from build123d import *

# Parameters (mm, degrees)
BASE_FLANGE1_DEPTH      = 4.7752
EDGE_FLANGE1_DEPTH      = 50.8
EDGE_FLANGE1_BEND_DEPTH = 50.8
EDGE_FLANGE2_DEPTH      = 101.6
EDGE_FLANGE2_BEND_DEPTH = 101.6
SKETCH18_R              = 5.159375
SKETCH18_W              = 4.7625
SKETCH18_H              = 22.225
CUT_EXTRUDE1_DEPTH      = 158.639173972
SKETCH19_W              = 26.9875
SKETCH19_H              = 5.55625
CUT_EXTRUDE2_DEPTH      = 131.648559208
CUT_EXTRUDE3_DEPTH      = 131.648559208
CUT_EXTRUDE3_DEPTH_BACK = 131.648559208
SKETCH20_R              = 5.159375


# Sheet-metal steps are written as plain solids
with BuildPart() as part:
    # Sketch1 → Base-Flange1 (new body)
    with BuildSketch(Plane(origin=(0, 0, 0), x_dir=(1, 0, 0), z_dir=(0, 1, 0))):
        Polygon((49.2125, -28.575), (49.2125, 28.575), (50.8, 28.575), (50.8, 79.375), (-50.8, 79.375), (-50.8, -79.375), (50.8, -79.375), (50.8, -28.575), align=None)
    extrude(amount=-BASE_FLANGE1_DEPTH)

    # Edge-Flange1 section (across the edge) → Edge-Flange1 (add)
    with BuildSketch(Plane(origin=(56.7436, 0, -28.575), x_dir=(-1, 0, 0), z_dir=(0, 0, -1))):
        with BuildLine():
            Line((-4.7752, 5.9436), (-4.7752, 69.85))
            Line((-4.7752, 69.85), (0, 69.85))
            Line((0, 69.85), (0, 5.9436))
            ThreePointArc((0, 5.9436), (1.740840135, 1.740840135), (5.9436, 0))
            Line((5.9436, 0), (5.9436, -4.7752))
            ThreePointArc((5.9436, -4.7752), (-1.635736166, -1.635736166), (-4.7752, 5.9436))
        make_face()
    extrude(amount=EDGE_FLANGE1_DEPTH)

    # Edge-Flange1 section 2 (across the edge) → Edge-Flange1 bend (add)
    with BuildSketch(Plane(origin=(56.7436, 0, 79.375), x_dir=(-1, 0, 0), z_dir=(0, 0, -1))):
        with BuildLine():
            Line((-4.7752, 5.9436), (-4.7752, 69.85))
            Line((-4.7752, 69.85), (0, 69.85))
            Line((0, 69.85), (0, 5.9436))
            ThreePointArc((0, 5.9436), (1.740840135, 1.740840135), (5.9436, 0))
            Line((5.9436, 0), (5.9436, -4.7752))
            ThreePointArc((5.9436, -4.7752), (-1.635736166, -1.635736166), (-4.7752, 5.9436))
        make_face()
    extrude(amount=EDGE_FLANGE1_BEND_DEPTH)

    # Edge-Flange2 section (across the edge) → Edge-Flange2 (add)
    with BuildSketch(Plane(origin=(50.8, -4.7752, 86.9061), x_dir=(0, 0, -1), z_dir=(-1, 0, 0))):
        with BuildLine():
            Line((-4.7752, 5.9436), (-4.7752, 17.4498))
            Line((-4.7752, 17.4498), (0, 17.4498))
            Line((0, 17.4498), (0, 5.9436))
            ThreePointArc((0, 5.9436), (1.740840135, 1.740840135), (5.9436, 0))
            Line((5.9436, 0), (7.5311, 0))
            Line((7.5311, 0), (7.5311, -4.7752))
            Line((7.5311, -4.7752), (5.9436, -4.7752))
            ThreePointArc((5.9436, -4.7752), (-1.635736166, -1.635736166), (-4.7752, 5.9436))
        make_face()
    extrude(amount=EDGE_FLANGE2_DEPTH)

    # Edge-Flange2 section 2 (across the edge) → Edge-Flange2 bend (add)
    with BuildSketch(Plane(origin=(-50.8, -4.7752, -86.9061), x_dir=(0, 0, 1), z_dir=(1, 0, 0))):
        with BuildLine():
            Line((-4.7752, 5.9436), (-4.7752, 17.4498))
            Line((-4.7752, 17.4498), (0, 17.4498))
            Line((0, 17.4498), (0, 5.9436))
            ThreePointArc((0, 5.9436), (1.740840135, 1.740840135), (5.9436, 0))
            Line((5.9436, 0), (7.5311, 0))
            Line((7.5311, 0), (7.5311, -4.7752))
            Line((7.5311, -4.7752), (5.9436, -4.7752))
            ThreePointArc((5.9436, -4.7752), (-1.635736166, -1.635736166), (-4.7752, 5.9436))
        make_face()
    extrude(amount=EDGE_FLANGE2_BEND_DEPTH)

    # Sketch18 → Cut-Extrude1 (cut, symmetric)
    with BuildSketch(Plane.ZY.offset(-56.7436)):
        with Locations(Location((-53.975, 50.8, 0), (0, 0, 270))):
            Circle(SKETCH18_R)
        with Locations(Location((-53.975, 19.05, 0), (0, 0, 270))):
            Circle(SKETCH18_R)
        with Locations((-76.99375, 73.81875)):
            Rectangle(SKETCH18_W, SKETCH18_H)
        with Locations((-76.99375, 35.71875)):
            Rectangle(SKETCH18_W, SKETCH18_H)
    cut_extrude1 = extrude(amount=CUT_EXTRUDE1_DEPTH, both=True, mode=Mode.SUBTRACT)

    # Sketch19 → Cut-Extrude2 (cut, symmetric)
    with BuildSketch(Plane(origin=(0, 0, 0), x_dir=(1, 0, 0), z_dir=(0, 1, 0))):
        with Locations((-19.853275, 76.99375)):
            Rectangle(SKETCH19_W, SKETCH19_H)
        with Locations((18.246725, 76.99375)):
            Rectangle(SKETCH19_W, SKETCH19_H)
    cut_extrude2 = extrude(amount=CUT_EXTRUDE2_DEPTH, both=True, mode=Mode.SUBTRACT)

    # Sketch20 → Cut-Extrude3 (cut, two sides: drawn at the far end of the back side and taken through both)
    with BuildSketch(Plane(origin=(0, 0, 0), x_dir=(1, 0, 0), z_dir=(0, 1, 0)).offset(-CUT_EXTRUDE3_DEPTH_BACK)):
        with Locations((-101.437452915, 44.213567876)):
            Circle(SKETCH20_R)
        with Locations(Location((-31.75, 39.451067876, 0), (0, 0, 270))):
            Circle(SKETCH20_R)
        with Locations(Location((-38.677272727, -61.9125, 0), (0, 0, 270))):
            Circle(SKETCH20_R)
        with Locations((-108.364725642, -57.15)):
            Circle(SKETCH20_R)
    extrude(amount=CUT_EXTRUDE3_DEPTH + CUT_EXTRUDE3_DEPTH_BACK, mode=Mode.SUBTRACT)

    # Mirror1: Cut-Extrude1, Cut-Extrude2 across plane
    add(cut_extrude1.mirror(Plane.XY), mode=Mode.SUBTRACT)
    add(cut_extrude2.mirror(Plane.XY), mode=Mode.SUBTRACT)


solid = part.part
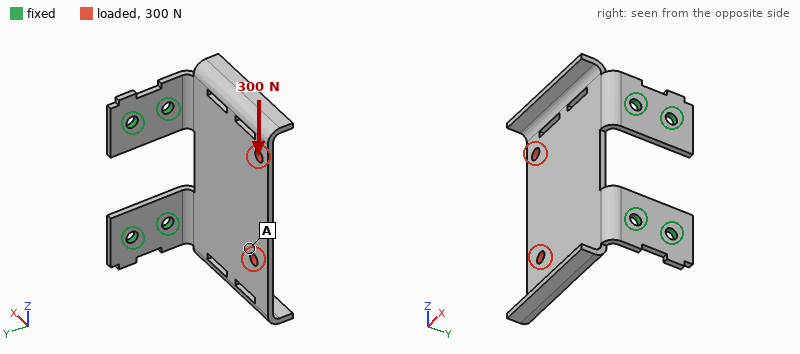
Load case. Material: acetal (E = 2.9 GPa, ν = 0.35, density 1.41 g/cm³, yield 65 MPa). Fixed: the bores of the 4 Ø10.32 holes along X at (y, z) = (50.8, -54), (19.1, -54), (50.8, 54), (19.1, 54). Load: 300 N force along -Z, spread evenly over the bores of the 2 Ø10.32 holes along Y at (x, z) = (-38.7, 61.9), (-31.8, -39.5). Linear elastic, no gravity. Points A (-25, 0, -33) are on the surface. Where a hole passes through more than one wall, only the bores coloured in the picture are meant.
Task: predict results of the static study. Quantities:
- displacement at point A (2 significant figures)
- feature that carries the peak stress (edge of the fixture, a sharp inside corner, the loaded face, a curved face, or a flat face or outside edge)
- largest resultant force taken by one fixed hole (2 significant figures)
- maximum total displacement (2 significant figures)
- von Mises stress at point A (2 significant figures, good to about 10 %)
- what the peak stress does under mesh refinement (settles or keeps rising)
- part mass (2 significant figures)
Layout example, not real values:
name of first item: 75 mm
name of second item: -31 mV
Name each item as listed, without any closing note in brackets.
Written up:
displacement at point A: 0.91 mm
feature that carries the peak stress: edge of the fixture
largest resultant force taken by one fixed hole: 340 N
maximum total displacement: 2.0 mm
von Mises stress at point A: 2.3 MPa
what the peak stress does under mesh refinement: keeps rising
part mass: 190 g
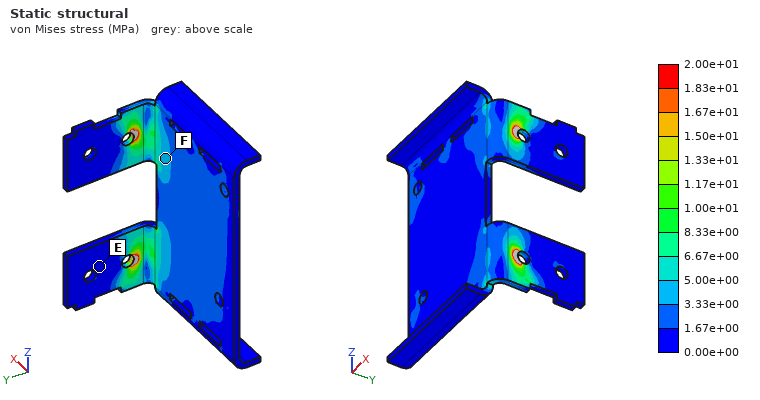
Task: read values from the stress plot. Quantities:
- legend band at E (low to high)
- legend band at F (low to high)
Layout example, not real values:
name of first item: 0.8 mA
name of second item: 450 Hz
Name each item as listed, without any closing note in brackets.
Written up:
legend band at E: 0.00e+00 to 1.67e+00 MPa
legend band at F: 3.33e+00 to 5.00e+00 MPa
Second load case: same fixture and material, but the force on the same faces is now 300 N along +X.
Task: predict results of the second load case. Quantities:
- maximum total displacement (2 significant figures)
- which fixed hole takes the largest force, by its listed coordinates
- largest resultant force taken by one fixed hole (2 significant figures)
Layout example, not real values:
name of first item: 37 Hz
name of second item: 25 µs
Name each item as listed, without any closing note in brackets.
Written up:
maximum total displacement: 2.7 mm
which fixed hole takes the largest force, by its listed coordinates: (19.1, 54)
largest resultant force taken by one fixed hole: 200 N
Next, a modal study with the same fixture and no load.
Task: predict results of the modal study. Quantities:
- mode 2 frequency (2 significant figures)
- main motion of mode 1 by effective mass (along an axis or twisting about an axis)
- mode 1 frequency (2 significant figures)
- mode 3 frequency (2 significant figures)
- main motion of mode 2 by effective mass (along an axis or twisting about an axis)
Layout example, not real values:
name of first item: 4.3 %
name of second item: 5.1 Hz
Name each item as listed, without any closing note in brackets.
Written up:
mode 2 frequency: 110 Hz
main motion of mode 1 by effective mass: along Y
mode 1 frequency: 59 Hz
mode 3 frequency: 260 Hz
main motion of mode 2 by effective mass: twisting about X
